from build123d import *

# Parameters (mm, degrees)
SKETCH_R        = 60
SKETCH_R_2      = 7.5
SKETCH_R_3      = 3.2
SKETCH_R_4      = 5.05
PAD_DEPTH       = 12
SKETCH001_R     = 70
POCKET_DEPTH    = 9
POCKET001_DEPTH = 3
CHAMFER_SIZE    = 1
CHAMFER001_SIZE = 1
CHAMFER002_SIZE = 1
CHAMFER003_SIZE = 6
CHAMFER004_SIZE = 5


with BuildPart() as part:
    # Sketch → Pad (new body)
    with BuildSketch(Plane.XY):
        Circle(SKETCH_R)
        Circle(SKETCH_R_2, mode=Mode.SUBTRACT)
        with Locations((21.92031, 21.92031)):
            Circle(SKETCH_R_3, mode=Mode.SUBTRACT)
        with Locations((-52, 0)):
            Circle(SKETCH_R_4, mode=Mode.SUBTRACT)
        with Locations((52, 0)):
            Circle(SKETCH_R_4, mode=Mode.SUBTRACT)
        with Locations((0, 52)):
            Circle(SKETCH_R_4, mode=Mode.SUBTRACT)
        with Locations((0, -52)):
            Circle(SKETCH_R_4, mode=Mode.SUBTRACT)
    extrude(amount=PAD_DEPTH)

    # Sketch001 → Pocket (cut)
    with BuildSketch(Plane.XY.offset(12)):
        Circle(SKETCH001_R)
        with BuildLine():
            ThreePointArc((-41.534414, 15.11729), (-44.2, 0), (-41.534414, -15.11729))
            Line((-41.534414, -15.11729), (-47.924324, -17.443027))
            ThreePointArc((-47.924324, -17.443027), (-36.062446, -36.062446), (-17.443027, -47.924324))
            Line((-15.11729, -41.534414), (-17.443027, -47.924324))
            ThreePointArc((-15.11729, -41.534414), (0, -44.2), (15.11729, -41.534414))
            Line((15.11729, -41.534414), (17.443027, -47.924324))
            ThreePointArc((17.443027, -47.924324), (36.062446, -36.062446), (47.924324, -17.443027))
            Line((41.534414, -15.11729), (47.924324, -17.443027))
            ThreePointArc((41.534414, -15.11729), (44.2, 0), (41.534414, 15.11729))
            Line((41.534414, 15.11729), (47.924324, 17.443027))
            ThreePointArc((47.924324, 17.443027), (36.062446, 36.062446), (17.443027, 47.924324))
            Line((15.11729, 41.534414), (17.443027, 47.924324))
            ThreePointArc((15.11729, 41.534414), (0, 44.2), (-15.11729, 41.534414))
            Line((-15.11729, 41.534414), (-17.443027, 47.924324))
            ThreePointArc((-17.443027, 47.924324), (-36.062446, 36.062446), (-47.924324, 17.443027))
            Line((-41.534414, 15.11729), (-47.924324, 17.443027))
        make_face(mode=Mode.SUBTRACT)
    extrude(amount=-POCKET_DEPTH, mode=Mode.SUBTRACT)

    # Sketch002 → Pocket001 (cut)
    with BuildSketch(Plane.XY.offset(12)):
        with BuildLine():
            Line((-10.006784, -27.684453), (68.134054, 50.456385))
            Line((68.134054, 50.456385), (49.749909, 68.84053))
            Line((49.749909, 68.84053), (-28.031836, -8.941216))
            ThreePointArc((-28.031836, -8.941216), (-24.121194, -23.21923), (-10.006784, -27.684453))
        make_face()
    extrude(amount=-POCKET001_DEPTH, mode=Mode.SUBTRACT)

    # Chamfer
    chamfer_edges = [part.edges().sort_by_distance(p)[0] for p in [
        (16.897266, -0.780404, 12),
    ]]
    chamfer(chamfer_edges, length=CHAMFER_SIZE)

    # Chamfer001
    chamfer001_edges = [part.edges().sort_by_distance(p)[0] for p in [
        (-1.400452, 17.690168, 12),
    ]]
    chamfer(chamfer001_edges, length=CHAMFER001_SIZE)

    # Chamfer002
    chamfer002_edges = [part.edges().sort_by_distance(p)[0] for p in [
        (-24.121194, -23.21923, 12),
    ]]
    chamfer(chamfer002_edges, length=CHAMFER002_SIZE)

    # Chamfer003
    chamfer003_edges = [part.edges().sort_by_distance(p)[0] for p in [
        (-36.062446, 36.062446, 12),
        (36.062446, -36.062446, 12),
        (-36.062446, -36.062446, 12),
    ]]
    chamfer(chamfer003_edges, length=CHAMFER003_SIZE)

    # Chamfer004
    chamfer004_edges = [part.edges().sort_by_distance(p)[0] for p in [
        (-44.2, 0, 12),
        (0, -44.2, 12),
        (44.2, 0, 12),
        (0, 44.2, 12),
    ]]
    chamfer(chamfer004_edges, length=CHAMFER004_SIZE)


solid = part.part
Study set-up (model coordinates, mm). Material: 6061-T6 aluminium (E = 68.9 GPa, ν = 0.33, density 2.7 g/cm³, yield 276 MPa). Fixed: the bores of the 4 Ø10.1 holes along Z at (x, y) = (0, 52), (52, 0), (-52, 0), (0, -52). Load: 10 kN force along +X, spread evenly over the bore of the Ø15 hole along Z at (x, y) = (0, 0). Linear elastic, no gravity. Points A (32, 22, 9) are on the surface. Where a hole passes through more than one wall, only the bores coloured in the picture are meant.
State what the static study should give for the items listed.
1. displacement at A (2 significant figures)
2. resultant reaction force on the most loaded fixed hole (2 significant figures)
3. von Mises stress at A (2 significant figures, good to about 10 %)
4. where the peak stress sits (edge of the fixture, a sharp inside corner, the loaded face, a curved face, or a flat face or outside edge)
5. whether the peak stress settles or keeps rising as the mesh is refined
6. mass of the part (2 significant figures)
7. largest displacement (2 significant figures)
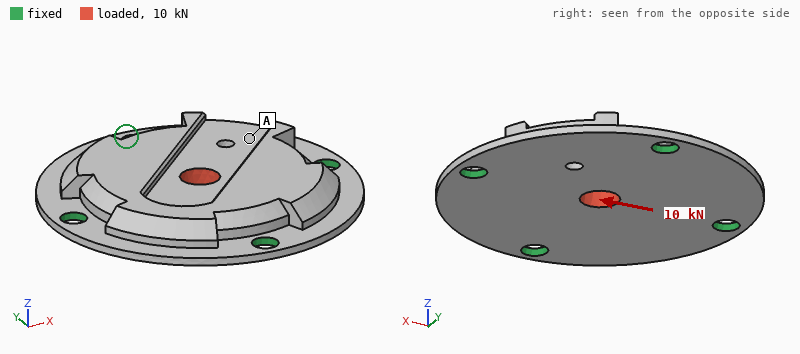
9.3 µm
3.1 kN
9.6 MPa
a sharp inside corner
keeps rising
230 g
16 µm
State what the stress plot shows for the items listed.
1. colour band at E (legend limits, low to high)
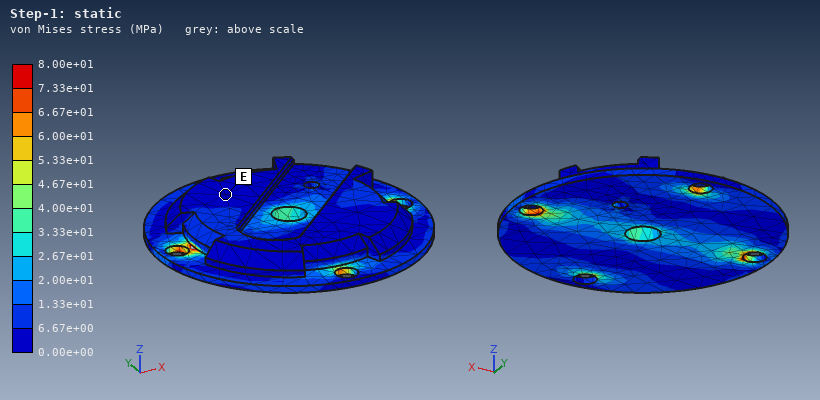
0.00e+00 to 6.67e+00 MPa
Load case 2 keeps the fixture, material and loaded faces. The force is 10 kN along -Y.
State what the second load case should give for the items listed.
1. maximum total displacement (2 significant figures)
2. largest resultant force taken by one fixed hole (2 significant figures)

16 µm
3.1 kN
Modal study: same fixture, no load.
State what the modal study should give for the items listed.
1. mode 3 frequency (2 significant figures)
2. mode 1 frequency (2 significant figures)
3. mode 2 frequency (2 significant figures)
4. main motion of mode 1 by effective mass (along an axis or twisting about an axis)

5900 Hz
4700 Hz
5600 Hz
along Z
